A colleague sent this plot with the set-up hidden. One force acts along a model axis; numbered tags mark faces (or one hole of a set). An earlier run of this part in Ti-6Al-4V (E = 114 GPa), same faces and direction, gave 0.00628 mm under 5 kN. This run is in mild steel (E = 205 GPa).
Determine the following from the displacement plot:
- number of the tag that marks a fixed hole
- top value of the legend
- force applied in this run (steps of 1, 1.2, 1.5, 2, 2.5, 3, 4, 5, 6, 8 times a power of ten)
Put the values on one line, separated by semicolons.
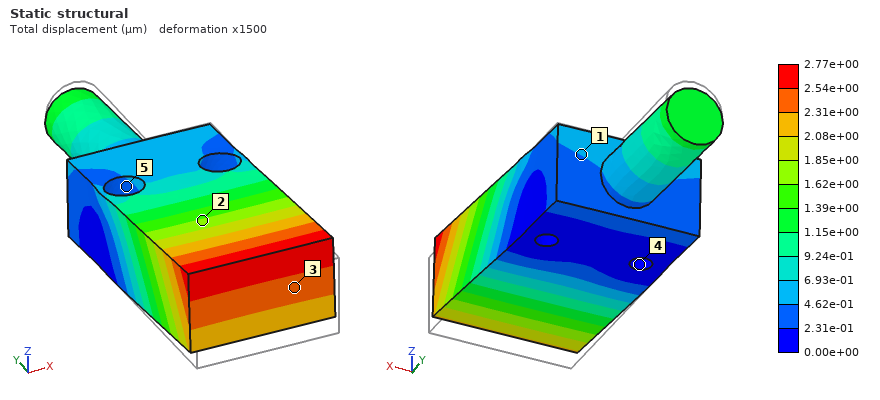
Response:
4; 2.77e+00 µm; 4 kN
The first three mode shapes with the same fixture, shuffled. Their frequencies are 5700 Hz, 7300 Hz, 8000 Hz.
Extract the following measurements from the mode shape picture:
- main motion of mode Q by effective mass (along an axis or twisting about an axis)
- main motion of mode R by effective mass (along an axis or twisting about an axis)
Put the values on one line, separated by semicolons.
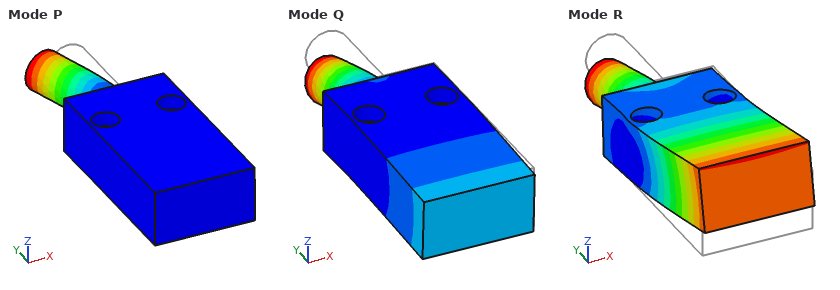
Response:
along Z; along Z
